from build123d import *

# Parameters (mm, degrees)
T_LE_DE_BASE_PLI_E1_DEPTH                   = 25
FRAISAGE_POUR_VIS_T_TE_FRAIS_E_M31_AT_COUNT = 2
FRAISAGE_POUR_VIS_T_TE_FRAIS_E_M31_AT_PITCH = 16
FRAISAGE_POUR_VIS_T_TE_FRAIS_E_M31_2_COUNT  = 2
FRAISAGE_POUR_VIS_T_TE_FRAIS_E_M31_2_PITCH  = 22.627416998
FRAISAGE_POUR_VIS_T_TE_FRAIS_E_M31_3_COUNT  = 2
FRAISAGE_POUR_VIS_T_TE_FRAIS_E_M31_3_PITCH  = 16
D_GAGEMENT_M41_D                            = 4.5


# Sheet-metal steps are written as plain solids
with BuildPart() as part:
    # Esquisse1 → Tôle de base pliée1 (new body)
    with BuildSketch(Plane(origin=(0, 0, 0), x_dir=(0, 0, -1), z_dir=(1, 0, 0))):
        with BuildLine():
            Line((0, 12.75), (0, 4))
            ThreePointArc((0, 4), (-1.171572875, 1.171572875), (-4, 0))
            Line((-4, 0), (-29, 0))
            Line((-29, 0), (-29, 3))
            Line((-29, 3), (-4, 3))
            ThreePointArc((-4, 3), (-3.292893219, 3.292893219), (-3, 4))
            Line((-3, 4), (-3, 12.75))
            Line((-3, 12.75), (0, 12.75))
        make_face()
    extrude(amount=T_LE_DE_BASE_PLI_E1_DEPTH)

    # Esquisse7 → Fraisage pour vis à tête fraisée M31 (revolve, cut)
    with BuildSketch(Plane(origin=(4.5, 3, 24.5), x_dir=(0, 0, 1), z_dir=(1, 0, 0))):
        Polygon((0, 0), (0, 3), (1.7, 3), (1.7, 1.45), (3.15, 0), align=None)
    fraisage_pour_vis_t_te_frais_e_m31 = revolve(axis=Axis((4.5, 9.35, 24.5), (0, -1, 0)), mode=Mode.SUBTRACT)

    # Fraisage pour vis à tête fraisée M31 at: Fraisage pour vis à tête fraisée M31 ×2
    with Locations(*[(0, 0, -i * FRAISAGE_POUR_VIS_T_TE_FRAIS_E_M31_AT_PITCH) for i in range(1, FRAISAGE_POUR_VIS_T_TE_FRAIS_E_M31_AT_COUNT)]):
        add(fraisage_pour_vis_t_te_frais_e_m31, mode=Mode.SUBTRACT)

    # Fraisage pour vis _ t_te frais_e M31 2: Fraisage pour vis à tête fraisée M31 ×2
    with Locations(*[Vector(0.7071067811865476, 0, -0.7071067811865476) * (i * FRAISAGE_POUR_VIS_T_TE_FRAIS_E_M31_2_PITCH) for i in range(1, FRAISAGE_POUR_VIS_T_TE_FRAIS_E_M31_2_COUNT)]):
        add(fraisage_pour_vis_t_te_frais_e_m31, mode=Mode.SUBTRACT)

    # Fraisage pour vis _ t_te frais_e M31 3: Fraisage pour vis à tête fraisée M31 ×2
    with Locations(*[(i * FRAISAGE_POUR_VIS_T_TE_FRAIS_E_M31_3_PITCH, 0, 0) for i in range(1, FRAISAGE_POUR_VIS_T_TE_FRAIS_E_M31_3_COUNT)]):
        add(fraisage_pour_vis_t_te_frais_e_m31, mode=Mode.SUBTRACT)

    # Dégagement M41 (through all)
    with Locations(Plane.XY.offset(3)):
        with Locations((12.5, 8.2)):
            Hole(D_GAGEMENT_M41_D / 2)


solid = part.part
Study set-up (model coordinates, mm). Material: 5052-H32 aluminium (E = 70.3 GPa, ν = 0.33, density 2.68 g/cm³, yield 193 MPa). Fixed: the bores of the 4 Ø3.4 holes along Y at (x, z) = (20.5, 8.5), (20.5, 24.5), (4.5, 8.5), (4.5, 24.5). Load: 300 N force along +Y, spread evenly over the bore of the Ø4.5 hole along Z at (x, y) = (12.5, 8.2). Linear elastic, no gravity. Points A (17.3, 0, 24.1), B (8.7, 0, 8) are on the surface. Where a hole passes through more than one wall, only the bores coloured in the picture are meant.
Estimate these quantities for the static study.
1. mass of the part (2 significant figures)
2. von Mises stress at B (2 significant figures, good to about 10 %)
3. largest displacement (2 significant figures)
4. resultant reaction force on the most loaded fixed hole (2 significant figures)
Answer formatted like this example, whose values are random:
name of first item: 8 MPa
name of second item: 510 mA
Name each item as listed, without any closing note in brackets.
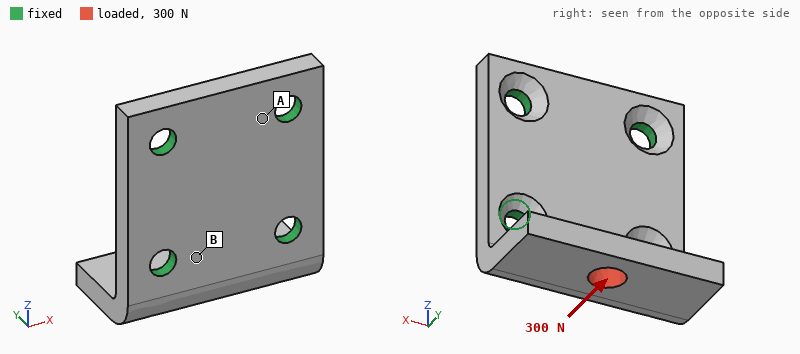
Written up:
mass of the part: 7.0 g
von Mises stress at B: 28 MPa
largest displacement: 36 µm
resultant reaction force on the most loaded fixed hole: 190 N
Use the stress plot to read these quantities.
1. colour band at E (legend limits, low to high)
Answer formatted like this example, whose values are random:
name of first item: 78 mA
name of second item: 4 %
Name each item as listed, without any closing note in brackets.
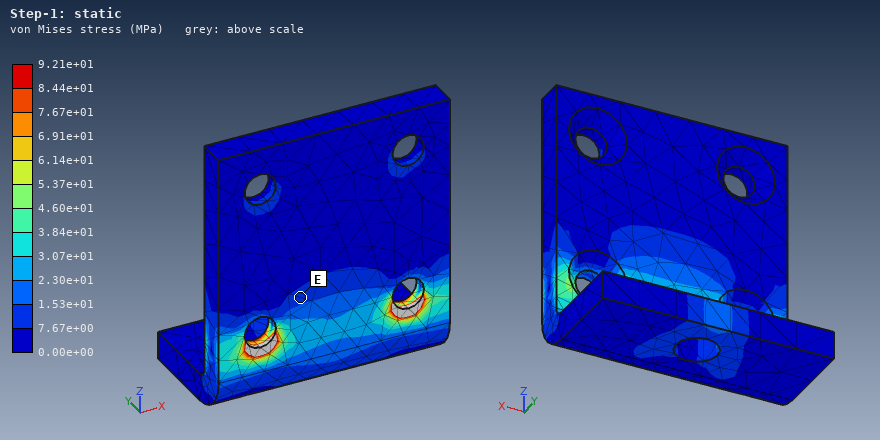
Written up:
colour band at E: 7.67e+00 to 1.53e+01 MPa
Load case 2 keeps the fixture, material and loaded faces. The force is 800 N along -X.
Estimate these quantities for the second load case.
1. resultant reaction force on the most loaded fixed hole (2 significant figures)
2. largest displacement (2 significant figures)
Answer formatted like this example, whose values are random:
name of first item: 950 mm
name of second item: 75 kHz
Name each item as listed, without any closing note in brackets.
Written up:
resultant reaction force on the most loaded fixed hole: 610 N
largest displacement: 41 µm
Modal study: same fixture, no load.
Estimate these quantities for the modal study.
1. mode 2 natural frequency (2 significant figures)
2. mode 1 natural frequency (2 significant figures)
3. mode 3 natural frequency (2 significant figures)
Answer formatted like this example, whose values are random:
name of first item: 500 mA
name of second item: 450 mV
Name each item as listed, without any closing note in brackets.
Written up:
mode 2 natural frequency: 15 kHz
mode 1 natural frequency: 8900 Hz
mode 3 natural frequency: 26 kHz
